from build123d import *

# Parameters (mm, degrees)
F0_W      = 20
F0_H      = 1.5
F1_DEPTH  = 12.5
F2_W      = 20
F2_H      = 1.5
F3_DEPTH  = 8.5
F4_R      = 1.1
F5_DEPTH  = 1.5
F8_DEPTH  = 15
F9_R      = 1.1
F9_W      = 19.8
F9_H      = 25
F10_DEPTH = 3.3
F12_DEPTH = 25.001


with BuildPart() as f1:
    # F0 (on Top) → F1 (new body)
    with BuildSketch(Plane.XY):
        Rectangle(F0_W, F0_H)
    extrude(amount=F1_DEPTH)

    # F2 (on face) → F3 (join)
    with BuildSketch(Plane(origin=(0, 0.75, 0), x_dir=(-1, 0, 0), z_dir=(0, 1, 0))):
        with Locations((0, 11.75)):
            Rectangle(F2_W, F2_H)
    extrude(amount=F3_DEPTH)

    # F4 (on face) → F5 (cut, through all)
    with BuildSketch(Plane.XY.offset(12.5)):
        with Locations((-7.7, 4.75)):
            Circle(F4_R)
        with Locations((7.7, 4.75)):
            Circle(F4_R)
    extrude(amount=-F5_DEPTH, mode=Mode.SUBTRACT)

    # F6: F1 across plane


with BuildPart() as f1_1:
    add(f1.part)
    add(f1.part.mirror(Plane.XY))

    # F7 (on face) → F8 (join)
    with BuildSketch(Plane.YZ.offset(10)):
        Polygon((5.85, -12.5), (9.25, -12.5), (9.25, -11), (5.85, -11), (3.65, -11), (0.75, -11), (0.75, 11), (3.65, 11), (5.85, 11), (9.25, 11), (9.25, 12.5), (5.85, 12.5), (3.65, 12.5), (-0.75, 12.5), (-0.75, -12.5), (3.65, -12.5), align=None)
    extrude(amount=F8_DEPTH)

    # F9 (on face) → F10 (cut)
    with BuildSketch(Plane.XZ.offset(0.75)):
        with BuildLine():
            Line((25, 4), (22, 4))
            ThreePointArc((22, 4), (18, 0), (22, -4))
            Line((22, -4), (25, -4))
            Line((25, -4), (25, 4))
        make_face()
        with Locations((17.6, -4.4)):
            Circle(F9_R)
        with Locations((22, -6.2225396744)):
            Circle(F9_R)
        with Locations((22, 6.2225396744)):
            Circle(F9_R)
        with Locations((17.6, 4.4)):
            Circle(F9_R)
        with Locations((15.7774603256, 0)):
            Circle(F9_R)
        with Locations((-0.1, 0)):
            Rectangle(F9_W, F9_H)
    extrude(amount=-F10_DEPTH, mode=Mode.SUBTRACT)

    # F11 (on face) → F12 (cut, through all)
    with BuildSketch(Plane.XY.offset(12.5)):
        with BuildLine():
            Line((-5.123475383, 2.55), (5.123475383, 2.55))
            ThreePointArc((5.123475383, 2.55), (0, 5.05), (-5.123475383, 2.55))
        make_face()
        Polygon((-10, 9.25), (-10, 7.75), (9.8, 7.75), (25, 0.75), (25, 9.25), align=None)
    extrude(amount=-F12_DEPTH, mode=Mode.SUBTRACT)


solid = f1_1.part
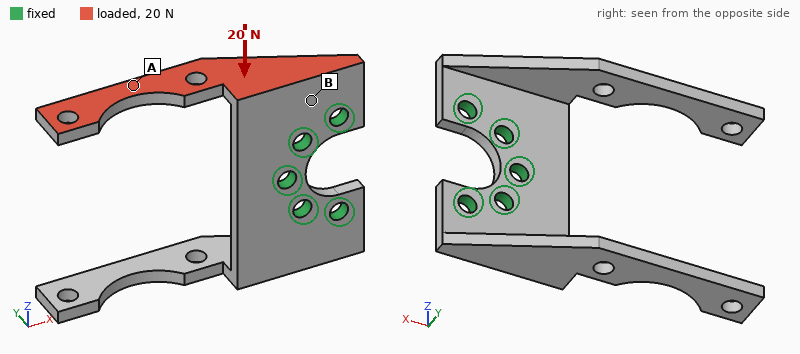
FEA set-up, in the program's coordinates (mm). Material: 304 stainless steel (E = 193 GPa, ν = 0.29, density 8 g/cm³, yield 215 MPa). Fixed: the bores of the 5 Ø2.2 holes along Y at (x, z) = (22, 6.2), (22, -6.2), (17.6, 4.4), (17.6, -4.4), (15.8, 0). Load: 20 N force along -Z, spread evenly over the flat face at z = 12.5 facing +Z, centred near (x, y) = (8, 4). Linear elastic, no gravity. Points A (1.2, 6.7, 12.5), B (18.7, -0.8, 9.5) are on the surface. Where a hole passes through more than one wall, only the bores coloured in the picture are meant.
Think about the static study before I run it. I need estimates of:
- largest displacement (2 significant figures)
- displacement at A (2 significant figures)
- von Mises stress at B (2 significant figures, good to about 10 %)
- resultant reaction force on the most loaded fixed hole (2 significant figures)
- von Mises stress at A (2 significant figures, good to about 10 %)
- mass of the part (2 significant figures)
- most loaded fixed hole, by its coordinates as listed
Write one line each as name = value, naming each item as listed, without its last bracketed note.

largest displacement = 0.10 mm
displacement at A = 0.042 mm
von Mises stress at B = 13 MPa
resultant reaction force on the most loaded fixed hole = 18 N
von Mises stress at A = 32 MPa
mass of the part = 6.9 g
most loaded fixed hole, by its coordinates as listed = (15.8, 0)
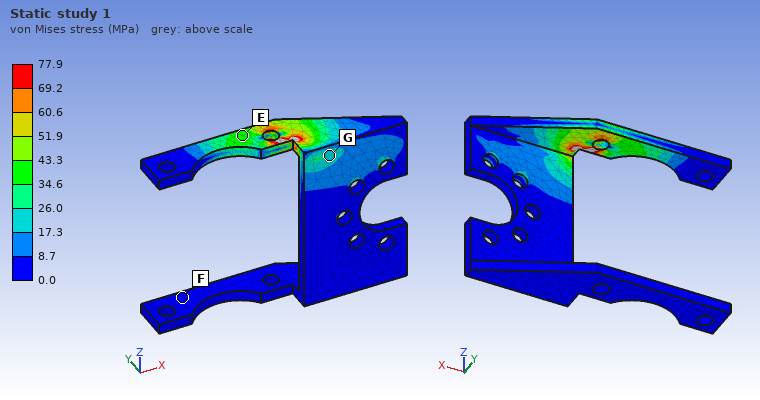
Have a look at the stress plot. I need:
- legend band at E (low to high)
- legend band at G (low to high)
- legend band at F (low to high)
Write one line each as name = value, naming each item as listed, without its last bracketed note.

legend band at E = 34.6 to 43.3 MPa
legend band at G = 17.3 to 26.0 MPa
legend band at F = 0.0 to 8.7 MPa
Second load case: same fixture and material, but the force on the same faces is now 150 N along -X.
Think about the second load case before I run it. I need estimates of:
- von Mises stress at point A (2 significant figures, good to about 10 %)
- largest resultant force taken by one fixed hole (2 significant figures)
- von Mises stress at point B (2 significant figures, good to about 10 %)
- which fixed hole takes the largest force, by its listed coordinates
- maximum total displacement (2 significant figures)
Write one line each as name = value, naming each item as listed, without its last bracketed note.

von Mises stress at point A = 34 MPa
largest resultant force taken by one fixed hole = 160 N
von Mises stress at point B = 38 MPa
which fixed hole takes the largest force, by its listed coordinates = (22, 6.2)
maximum total displacement = 76 µm
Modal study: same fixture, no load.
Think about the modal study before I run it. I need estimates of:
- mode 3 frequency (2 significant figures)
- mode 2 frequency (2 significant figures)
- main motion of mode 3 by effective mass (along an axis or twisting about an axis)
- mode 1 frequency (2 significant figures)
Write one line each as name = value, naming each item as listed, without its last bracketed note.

mode 3 frequency = 3400 Hz
mode 2 frequency = 2000 Hz
main motion of mode 3 by effective mass = twisting about X
mode 1 frequency = 2000 Hz
